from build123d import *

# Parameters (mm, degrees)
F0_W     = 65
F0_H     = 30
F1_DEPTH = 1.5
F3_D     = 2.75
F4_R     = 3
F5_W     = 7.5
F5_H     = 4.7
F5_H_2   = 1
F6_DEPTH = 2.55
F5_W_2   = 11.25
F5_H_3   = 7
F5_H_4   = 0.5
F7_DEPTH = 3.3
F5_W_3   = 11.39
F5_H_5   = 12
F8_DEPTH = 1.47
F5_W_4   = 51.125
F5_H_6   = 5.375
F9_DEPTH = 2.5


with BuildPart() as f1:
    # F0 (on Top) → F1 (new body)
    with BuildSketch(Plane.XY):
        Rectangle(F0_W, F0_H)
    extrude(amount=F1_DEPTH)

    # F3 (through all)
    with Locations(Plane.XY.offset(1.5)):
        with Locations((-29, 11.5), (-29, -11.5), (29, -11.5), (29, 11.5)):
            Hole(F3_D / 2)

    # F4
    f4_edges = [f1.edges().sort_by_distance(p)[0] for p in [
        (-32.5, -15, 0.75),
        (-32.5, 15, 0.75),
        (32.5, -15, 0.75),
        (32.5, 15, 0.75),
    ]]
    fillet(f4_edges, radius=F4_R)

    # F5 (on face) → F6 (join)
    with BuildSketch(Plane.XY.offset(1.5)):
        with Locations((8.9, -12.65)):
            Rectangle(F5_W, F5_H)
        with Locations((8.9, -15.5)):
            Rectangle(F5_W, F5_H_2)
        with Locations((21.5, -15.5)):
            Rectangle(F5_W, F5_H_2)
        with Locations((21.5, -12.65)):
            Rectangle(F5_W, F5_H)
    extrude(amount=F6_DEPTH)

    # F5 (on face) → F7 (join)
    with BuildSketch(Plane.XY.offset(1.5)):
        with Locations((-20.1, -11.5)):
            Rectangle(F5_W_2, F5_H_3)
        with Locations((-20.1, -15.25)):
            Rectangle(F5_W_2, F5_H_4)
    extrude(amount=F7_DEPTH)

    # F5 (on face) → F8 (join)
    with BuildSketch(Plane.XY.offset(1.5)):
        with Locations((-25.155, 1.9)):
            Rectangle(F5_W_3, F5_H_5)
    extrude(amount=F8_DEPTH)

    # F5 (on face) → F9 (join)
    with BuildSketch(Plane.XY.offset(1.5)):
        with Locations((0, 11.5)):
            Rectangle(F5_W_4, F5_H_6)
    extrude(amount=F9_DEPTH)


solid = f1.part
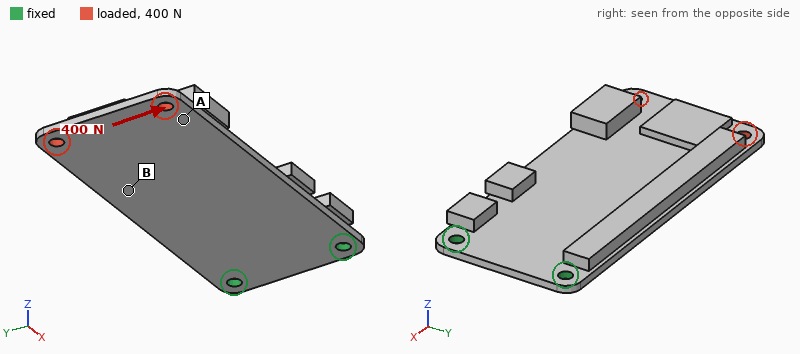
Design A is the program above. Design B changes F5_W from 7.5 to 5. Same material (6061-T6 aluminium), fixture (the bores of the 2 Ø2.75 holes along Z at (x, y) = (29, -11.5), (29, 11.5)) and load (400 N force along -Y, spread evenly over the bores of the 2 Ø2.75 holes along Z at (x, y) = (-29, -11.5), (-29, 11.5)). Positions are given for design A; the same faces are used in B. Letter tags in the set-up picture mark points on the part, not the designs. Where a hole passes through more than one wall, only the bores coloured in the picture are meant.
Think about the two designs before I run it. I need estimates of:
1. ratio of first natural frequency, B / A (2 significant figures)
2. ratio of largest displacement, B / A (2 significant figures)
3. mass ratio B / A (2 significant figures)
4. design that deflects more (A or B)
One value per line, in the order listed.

0.97
1.1
0.98
B
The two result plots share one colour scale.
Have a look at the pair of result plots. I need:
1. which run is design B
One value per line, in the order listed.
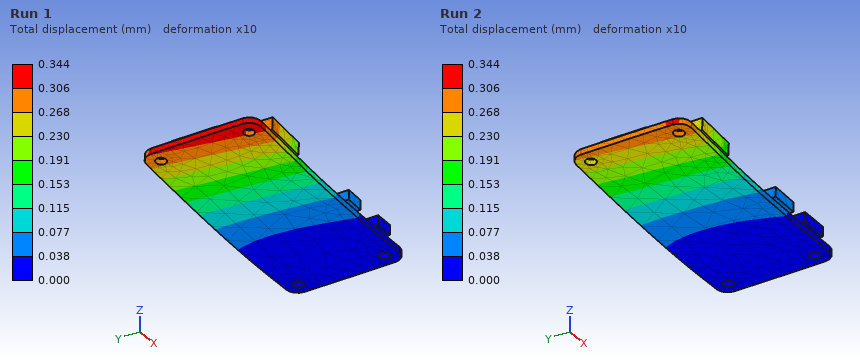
Run 1
